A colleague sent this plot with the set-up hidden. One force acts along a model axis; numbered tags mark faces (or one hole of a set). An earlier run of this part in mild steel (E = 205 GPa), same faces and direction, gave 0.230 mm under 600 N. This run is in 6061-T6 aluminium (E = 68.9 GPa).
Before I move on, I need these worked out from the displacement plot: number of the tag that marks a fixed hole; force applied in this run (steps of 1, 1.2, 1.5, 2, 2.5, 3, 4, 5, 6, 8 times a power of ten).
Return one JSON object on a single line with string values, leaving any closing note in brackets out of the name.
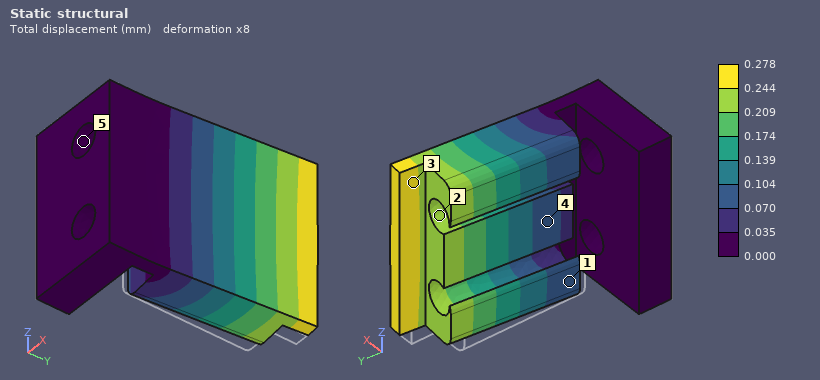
{"number of the tag that marks a fixed hole": "5", "force applied in this run": "250 N"}
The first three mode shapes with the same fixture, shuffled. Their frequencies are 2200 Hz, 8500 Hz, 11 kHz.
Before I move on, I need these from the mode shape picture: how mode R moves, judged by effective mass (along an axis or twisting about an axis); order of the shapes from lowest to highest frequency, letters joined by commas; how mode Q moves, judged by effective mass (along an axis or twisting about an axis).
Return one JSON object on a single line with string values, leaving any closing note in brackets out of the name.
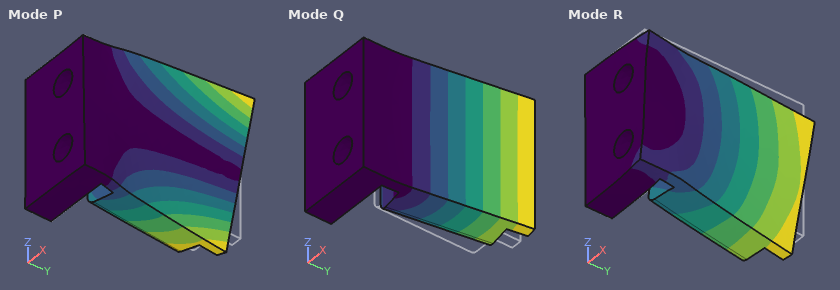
{"how mode R moves, judged by effective mass": "along Z", "order of the shapes from lowest to highest frequency, letters joined by commas": "Q, P, R", "how mode Q moves, judged by effective mass": "along X"}
